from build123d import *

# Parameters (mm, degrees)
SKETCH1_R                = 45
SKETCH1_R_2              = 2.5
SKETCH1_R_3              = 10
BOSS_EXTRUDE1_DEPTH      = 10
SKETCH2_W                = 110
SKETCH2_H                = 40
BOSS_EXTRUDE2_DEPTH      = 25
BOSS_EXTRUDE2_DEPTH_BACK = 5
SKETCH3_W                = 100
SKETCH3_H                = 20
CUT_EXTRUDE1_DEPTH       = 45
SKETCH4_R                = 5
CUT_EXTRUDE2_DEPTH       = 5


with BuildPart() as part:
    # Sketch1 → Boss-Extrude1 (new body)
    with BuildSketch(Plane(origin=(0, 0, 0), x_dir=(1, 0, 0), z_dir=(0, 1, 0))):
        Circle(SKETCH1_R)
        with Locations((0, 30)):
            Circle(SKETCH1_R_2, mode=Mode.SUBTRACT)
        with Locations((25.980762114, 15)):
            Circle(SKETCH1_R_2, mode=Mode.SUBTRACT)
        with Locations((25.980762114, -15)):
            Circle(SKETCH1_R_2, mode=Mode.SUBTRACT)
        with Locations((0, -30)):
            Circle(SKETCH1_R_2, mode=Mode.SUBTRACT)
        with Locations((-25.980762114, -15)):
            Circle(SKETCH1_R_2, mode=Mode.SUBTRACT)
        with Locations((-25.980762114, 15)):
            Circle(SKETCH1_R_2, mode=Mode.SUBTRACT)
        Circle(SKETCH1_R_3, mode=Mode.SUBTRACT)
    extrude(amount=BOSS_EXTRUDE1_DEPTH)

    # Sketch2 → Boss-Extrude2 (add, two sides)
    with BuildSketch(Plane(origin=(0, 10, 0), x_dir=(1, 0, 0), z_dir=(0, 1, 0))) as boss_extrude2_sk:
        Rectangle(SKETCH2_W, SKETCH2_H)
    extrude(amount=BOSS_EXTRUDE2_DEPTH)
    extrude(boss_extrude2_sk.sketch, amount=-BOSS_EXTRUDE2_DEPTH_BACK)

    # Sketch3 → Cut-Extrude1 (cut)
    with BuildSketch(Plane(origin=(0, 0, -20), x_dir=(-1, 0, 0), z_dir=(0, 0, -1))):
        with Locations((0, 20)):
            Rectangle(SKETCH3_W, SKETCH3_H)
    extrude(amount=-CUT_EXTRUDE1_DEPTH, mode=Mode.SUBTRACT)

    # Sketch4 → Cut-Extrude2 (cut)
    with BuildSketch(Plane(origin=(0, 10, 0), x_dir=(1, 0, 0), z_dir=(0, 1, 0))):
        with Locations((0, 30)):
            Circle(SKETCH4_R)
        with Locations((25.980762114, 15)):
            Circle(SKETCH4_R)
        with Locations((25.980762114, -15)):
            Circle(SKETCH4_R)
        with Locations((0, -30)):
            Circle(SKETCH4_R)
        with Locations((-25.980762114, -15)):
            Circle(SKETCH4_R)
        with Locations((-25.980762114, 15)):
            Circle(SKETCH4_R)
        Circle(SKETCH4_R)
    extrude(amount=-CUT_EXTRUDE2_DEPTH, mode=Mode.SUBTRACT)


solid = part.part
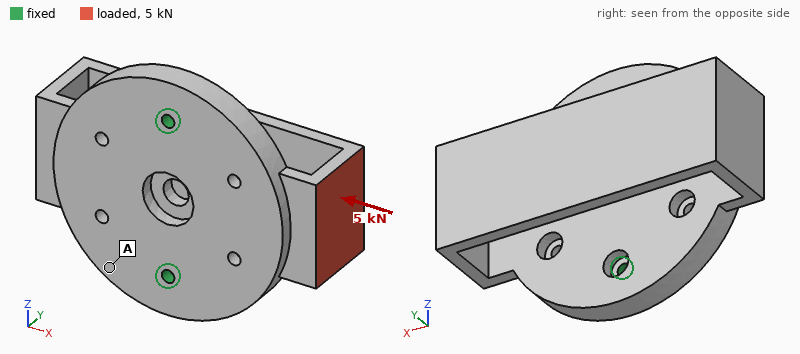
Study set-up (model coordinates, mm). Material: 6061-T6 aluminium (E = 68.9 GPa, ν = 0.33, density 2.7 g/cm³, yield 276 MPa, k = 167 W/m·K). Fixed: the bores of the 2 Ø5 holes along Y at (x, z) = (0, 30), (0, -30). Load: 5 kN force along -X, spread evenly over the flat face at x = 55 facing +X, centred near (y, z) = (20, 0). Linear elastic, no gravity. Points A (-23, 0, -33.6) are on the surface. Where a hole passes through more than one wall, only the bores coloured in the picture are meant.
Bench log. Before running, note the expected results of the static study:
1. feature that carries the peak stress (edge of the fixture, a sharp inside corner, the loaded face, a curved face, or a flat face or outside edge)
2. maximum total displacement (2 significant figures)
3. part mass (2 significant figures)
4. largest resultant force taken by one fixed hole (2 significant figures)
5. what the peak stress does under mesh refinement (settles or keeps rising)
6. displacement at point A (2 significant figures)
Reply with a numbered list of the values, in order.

1. edge of the fixture
2. 0.76 mm
3. 250 g
4. 2.5 kN
5. keeps rising
6. 0.14 mm
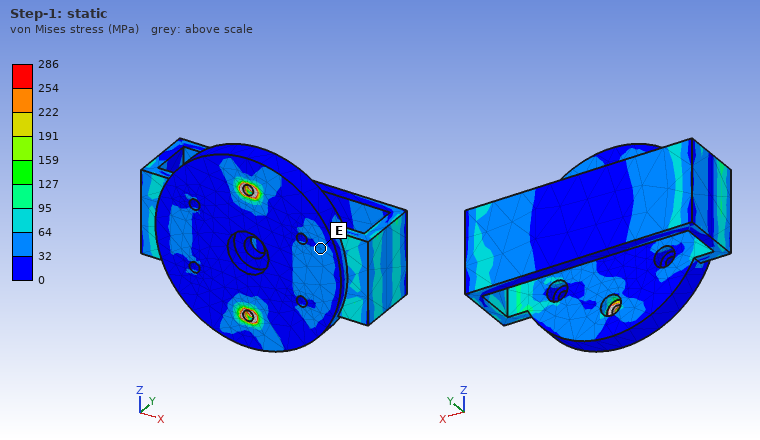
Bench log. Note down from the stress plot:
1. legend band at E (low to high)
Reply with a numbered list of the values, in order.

1. 32 to 64 MPa
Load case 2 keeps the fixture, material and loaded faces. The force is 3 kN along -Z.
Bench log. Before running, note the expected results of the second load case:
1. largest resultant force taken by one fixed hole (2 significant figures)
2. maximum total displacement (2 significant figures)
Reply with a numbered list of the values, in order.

1. 3.2 kN
2. 0.20 mm
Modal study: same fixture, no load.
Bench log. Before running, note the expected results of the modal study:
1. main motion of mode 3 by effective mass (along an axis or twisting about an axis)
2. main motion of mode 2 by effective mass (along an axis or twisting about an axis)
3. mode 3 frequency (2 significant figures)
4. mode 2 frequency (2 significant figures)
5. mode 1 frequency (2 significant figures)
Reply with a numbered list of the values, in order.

1. along Z
2. along Y
3. 2200 Hz
4. 1500 Hz
5. 960 Hz
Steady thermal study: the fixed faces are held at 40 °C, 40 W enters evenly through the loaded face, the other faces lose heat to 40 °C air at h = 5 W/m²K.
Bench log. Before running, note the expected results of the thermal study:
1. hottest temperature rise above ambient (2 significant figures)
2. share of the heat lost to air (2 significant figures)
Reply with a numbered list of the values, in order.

1. 37 K
2. 5.6 %
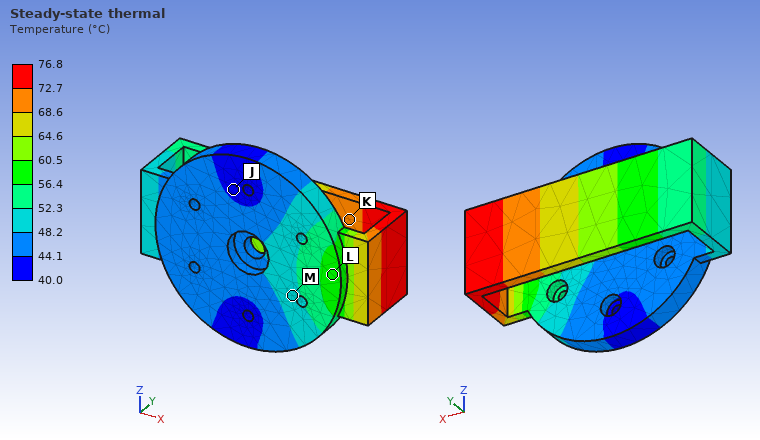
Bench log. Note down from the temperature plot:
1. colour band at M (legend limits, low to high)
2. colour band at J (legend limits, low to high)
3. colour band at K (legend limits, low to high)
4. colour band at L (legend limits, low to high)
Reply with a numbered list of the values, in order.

1. 48.2 to 52.3 °C
2. 40.0 to 44.1 °C
3. 68.6 to 72.7 °C
4. 56.4 to 60.5 °C
